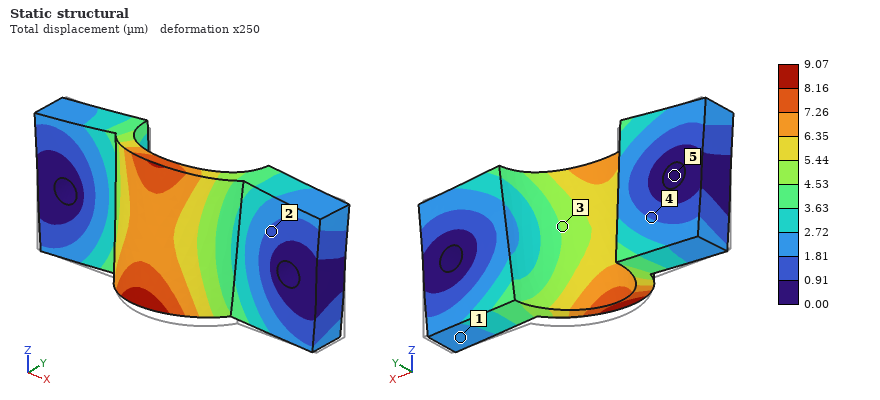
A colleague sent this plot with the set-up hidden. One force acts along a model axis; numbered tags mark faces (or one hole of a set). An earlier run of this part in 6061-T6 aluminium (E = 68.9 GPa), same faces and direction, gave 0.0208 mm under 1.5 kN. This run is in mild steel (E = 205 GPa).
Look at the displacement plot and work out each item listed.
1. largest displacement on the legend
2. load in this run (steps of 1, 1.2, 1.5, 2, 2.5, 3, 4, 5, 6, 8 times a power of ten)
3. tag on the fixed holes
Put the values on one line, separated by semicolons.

9.07 µm; 2 kN; 5
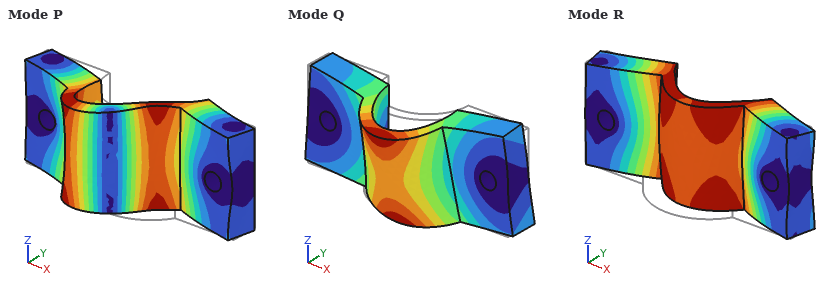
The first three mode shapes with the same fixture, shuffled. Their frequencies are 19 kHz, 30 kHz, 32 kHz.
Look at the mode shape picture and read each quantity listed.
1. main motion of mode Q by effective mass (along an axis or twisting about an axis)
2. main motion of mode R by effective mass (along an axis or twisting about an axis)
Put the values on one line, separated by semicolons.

along Z; along Y
